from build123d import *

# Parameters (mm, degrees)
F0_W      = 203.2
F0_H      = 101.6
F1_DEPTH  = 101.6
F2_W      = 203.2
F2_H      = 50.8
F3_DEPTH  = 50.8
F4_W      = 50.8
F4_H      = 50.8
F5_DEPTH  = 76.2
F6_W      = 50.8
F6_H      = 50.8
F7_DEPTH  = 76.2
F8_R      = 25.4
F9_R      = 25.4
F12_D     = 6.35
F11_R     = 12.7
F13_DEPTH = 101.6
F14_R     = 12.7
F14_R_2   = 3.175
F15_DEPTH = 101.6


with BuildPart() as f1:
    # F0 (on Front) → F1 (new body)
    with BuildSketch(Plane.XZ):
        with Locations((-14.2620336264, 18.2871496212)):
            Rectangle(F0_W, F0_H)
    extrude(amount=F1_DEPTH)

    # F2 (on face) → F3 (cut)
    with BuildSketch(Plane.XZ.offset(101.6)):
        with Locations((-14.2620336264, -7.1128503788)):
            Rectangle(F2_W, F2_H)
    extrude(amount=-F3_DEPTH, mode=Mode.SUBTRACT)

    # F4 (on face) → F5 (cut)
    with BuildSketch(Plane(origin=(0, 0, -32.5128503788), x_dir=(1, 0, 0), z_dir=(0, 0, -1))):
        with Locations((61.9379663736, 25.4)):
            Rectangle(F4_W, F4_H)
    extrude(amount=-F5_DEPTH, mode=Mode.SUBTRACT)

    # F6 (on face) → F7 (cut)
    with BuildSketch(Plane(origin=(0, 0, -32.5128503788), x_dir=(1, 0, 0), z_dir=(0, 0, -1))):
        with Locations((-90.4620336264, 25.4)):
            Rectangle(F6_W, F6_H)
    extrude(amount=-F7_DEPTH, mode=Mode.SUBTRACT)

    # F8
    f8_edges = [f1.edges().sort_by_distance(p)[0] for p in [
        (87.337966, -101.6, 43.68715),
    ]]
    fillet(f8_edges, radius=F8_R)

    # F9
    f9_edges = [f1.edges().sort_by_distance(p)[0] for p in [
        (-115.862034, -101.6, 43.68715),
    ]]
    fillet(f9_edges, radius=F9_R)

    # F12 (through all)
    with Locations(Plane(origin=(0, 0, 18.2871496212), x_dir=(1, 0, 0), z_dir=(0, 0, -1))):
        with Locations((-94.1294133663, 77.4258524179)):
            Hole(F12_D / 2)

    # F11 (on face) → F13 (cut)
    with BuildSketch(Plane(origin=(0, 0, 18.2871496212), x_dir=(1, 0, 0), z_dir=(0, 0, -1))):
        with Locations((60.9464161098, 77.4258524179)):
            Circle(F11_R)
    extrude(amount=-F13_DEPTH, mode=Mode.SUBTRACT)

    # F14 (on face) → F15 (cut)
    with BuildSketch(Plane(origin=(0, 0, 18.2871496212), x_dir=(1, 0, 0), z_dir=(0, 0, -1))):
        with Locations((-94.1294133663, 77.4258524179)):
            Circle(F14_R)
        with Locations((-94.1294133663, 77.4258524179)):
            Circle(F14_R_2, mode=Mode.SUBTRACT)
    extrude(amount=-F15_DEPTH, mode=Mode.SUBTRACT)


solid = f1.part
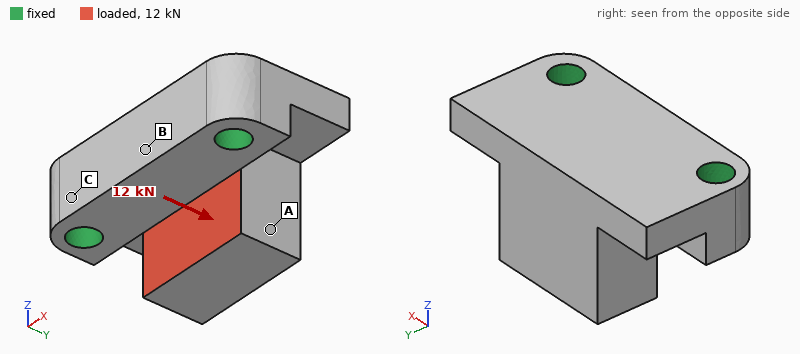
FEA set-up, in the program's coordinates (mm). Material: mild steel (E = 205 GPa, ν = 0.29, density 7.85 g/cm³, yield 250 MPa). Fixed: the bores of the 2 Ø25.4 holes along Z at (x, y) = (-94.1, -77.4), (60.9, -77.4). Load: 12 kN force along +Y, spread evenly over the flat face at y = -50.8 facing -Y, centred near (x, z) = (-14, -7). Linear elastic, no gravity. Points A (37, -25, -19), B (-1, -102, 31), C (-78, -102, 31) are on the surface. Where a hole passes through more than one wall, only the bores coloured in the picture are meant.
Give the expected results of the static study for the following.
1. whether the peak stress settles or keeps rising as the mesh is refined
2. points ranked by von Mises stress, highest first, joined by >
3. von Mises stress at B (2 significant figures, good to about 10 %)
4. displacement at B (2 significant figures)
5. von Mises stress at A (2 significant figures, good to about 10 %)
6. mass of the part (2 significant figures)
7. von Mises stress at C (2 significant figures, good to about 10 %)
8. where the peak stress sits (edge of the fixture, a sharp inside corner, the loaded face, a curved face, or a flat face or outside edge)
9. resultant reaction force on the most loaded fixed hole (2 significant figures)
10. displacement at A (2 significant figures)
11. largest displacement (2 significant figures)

keeps rising
C > B > A
4.3 MPa
4.0 µm
2.5 MPa
8.7 kg
9.1 MPa
a sharp inside corner
6.7 kN
15 µm
20 µm
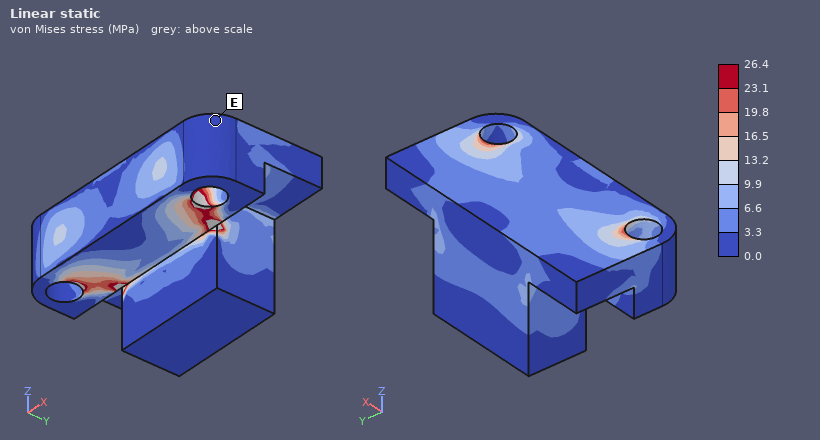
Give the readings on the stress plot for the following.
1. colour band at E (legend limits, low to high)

0.0 to 3.3 MPa
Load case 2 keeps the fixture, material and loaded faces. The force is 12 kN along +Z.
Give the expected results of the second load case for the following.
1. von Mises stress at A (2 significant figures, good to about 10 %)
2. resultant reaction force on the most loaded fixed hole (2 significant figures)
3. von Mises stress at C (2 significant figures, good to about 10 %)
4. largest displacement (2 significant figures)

1.7 MPa
6.2 kN
1.9 MPa
4.7 µm
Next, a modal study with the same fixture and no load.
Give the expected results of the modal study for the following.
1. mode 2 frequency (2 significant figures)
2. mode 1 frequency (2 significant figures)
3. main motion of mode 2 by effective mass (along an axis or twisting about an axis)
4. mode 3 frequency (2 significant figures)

4700 Hz
2400 Hz
along X
5400 Hz
